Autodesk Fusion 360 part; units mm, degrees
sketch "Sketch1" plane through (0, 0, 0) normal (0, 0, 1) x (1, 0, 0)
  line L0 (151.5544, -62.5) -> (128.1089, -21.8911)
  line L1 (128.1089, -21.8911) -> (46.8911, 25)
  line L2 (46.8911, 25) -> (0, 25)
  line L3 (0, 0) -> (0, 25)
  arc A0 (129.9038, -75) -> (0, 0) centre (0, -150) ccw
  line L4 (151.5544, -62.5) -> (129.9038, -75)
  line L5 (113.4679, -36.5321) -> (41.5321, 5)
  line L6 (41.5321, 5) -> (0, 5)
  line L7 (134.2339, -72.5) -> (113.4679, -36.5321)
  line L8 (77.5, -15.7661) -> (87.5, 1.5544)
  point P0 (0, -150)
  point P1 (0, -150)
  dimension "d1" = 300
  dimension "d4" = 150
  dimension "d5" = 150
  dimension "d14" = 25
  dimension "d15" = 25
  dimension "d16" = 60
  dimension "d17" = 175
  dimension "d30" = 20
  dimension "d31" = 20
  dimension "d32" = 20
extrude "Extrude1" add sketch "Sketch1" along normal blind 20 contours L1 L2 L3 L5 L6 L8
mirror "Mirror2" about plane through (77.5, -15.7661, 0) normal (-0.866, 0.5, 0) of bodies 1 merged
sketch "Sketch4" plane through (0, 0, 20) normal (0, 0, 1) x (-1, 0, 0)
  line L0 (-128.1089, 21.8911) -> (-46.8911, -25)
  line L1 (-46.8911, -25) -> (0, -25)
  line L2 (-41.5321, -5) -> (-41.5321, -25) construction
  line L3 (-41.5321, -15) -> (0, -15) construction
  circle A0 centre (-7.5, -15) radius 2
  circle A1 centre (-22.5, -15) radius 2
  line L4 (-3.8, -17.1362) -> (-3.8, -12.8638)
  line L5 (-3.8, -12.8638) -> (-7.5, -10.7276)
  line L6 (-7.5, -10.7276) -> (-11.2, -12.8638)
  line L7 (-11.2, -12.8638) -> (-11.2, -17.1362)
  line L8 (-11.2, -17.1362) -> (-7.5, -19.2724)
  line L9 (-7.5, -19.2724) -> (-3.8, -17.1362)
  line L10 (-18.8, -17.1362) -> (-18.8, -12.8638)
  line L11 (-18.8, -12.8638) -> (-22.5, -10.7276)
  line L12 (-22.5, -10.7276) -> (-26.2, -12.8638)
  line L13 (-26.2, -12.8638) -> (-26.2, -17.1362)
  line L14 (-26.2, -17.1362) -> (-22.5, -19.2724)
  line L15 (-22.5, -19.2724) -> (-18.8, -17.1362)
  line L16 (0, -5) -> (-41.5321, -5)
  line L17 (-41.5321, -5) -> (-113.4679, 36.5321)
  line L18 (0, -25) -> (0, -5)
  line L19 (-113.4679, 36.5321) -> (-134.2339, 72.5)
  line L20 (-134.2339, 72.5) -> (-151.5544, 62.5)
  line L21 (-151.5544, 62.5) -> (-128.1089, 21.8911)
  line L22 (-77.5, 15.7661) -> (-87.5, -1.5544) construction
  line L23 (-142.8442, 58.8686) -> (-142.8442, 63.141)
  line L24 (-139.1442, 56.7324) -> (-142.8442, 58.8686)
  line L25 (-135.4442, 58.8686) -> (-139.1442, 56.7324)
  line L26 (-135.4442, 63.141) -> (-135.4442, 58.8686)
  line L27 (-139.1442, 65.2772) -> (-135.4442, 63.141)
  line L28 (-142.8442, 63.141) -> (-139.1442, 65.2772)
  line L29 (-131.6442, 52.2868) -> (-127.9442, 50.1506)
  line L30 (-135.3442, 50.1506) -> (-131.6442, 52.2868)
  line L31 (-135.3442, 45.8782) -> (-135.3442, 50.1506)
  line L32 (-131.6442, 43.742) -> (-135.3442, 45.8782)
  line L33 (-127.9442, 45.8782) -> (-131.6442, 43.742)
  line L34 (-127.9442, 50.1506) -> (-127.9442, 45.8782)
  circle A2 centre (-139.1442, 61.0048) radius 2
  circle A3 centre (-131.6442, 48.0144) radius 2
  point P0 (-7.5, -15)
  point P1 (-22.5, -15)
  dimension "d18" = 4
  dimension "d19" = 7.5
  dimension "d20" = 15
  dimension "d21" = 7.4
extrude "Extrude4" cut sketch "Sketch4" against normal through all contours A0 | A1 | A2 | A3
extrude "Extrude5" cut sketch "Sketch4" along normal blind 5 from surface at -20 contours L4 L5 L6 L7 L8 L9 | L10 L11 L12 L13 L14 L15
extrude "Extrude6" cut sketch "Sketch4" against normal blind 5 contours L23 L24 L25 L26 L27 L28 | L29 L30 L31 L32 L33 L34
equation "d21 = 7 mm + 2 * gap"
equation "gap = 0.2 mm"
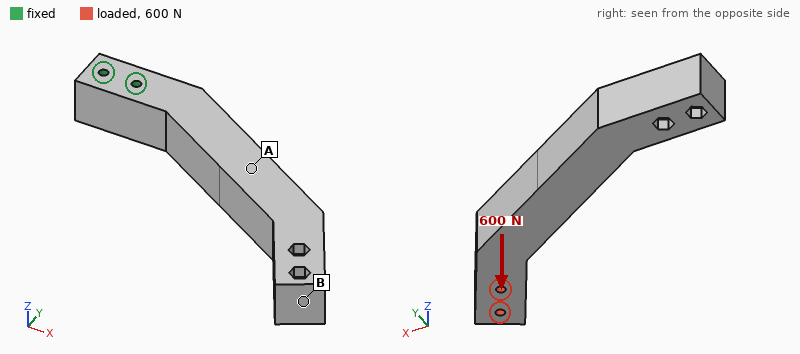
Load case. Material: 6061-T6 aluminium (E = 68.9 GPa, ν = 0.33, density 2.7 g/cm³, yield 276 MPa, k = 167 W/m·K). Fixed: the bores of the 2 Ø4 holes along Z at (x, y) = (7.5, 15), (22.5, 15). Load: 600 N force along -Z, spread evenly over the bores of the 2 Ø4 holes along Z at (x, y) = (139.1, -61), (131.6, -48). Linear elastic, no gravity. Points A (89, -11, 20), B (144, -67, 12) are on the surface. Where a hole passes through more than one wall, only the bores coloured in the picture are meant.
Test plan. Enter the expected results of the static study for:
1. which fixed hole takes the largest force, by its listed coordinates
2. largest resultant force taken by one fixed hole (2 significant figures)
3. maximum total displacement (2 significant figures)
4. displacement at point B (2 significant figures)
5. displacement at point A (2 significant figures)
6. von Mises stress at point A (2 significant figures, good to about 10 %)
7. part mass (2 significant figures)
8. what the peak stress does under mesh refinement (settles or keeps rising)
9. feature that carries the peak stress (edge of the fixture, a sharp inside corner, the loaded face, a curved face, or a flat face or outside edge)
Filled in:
(22.5, 15)
2.2 kN
0.80 mm
0.78 mm
0.26 mm
29 MPa
190 g
keeps rising
edge of the fixture
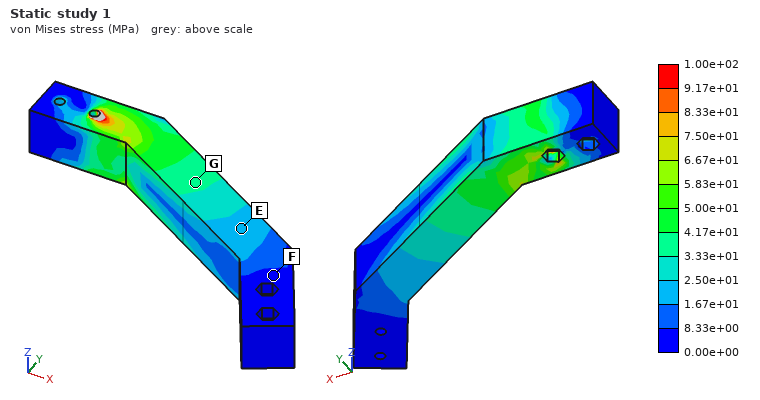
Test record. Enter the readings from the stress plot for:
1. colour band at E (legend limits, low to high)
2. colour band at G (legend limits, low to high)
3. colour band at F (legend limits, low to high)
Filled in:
1.67e+01 to 2.50e+01 MPa
3.33e+01 to 4.17e+01 MPa
0.00e+00 to 8.33e+00 MPa
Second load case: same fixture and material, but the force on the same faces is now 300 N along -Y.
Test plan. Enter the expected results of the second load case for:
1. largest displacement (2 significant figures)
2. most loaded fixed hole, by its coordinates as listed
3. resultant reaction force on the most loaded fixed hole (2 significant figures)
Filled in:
0.32 mm
(22.5, 15)
1.9 kN
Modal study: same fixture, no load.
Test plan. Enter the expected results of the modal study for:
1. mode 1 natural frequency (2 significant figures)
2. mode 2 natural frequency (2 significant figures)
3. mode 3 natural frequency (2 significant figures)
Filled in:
630 Hz
640 Hz
3200 Hz
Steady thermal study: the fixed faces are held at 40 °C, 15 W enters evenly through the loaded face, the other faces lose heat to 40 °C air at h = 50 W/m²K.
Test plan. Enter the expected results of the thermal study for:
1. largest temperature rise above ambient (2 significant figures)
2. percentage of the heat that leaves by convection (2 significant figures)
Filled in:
21 K
47 %
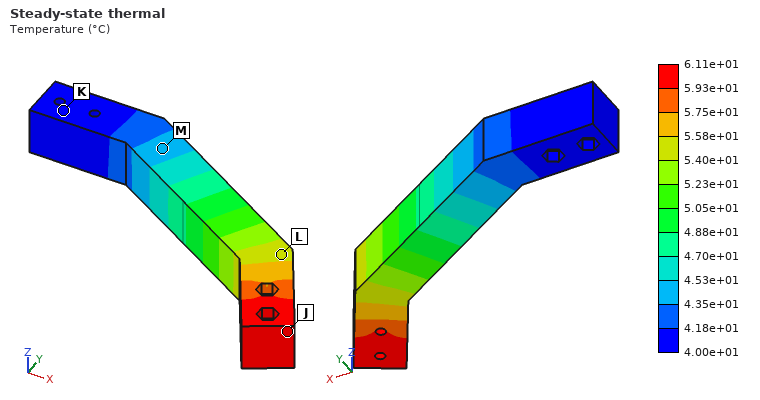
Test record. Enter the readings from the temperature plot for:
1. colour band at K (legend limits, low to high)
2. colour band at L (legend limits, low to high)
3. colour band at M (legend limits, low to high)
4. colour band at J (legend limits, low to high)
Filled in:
4.00e+01 to 4.18e+01 °C
5.40e+01 to 5.58e+01 °C
4.35e+01 to 4.53e+01 °C
5.93e+01 to 6.11e+01 °C
